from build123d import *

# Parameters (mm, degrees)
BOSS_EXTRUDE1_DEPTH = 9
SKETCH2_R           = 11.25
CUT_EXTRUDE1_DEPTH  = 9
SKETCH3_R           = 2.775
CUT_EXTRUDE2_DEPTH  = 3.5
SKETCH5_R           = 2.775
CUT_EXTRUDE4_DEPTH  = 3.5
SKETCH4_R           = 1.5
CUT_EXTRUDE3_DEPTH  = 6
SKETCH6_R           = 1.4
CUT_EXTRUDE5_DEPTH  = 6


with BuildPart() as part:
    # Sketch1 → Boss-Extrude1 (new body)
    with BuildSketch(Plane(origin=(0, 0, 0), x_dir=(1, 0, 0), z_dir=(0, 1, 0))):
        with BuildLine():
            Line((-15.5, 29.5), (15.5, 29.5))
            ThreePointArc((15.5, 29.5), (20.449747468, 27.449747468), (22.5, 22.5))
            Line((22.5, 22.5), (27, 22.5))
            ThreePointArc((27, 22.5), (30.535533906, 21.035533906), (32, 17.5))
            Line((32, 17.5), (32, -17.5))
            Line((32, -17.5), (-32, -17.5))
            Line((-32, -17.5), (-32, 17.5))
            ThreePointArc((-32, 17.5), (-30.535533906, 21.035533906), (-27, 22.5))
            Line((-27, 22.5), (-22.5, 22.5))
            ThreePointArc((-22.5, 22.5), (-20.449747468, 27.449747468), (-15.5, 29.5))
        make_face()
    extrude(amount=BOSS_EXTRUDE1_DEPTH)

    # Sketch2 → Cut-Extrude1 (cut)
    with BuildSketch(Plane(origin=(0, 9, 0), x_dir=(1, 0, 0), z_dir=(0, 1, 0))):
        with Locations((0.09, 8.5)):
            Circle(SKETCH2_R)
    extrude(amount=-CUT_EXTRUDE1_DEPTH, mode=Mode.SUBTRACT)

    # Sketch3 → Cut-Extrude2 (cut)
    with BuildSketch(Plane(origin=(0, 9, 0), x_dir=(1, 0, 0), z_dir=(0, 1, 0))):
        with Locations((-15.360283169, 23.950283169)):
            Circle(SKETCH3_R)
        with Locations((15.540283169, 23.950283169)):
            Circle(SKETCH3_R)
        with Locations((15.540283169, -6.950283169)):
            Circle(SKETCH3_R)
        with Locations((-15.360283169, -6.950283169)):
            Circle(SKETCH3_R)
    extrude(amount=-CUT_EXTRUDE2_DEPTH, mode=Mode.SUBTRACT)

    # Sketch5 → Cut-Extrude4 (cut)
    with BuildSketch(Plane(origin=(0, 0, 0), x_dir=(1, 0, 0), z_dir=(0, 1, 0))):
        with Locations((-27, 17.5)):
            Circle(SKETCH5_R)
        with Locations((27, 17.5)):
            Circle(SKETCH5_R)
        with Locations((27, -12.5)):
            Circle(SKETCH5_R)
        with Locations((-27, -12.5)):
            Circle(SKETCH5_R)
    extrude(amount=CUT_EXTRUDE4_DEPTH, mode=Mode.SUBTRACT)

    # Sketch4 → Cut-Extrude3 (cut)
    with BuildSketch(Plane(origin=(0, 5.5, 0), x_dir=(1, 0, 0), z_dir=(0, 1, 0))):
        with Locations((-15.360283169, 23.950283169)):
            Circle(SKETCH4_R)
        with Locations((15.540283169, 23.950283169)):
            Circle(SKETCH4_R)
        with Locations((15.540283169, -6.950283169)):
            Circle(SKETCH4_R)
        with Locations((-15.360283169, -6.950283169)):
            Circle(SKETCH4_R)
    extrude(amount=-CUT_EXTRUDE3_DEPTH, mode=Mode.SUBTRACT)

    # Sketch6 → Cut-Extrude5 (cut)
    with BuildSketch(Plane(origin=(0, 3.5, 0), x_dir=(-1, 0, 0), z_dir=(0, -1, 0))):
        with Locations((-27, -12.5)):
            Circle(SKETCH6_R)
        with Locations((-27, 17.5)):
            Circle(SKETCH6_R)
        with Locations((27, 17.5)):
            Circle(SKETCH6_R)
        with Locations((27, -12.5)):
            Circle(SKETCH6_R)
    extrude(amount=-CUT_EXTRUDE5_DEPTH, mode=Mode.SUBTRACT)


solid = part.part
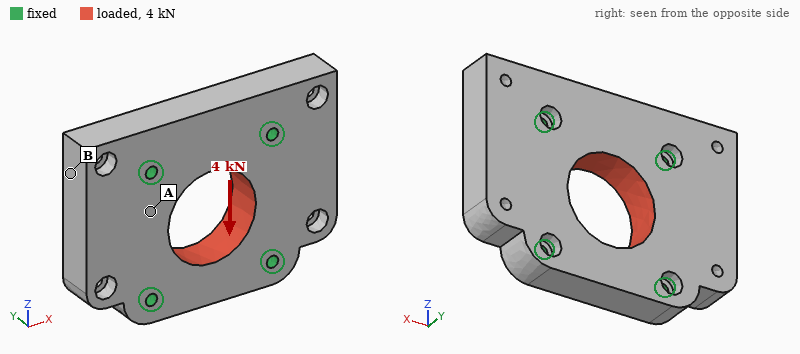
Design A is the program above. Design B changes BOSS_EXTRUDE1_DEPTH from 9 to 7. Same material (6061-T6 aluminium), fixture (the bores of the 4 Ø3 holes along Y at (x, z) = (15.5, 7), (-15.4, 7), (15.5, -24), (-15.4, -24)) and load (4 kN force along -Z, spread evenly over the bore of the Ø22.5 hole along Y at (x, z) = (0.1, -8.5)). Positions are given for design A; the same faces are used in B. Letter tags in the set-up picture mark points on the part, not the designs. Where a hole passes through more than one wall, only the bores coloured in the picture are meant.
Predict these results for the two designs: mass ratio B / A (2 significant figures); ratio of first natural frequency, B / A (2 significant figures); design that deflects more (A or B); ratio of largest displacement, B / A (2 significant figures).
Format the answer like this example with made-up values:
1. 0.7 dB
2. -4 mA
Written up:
1. 0.78
2. 0.95
3. B
4. 1.1
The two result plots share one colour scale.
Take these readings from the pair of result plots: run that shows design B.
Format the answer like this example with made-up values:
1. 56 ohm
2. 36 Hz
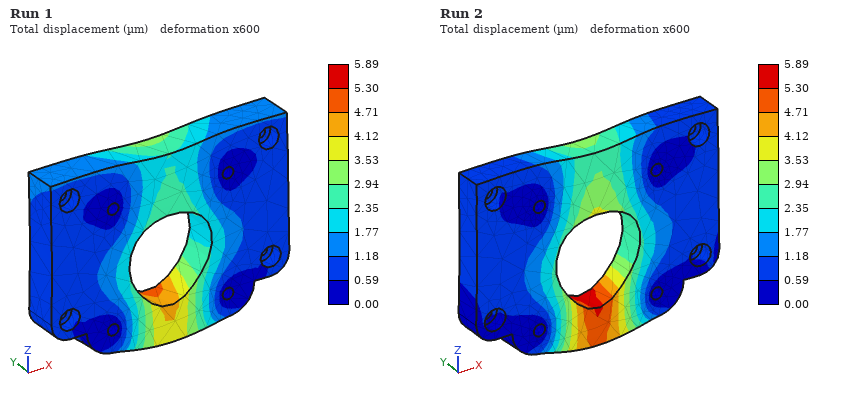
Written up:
1. Run 2
